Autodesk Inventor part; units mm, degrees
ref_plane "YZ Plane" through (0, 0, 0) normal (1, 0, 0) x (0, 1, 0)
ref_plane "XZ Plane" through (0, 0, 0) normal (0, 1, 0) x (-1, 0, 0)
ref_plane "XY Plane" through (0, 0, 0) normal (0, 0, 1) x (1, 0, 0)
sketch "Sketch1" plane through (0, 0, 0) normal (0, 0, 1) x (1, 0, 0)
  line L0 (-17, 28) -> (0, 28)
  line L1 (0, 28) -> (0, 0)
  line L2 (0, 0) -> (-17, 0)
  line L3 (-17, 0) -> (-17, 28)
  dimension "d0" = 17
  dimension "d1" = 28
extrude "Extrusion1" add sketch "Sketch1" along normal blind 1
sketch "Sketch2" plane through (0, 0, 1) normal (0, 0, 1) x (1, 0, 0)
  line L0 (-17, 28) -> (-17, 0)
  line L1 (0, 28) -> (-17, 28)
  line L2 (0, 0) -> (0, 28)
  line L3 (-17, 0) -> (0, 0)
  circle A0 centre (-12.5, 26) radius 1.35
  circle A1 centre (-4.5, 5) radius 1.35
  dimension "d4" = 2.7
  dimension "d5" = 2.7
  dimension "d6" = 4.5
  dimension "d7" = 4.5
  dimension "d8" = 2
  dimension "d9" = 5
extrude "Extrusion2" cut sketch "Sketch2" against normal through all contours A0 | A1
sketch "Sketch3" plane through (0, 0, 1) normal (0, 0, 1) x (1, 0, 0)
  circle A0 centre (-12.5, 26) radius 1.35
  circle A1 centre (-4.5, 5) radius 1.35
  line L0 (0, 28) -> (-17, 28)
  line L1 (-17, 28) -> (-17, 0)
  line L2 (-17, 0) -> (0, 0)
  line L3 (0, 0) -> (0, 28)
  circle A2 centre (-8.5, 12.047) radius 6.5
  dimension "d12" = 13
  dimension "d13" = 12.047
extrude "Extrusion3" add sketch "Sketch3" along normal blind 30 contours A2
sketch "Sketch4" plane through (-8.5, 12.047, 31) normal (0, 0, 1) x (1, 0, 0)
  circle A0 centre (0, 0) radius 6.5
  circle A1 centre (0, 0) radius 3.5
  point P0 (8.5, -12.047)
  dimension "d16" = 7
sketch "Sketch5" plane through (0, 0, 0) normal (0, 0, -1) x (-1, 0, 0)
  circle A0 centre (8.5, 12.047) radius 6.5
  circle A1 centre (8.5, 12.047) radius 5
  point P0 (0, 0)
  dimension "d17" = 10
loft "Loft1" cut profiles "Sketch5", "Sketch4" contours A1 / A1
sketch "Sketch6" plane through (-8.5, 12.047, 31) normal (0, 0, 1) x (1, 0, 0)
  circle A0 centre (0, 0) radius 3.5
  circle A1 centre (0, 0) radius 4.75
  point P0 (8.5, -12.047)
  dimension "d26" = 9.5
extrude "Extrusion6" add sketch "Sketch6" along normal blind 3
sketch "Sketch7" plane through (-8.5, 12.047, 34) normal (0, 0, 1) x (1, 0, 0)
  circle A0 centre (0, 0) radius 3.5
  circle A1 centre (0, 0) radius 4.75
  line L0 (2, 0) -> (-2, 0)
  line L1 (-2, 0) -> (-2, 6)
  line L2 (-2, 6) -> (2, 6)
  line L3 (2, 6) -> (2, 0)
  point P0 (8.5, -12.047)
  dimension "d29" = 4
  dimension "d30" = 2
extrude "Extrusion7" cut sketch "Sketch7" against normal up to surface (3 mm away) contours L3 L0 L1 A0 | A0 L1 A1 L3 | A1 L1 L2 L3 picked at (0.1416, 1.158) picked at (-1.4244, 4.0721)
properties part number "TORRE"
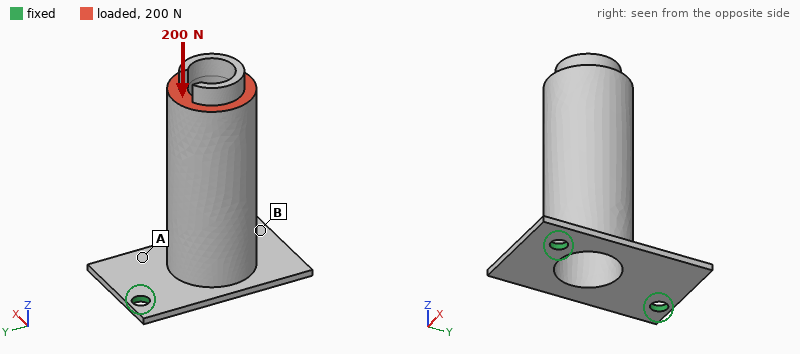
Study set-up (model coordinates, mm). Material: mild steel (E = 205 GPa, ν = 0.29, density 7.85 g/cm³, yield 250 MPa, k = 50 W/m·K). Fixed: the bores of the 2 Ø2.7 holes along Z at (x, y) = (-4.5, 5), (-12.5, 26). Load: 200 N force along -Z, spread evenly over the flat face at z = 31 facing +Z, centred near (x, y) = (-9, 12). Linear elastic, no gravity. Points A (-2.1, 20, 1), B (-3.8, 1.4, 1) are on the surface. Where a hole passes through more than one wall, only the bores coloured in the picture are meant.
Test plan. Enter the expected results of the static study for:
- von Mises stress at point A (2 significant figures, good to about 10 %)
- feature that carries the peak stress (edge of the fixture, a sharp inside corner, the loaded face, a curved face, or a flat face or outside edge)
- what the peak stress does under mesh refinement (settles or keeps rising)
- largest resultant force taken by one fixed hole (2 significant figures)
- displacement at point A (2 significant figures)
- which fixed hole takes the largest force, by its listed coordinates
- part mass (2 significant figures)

34 MPa
edge of the fixture
keeps rising
130 N
8.3 µm
(-4.5, 5)
22 g
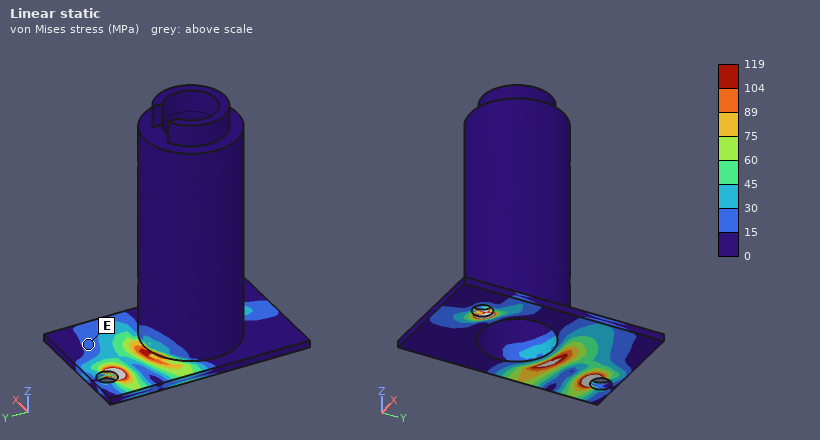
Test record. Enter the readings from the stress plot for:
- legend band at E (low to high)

15 to 30 MPa
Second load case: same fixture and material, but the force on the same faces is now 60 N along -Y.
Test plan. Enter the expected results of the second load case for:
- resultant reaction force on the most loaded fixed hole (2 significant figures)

95 N
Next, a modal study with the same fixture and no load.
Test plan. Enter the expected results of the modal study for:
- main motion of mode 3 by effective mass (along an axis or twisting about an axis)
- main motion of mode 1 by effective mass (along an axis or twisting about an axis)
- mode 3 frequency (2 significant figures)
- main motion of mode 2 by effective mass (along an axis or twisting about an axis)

along Z
along X
11 kHz
along Y
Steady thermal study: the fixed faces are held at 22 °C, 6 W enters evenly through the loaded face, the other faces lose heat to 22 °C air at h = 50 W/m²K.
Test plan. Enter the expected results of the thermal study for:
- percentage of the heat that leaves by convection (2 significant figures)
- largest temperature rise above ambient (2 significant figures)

56 %
45 K
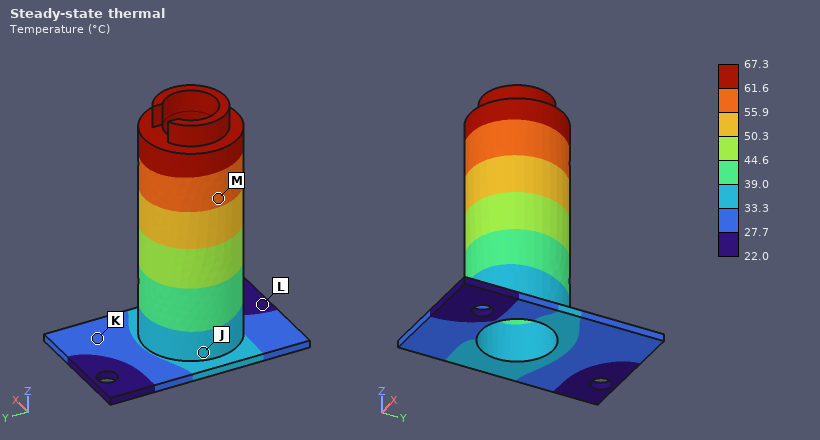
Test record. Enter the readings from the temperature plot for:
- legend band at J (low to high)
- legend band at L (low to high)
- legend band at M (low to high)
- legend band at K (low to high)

33.3 to 39.0 °C
22.0 to 27.7 °C
55.9 to 61.6 °C
27.7 to 33.3 °C
